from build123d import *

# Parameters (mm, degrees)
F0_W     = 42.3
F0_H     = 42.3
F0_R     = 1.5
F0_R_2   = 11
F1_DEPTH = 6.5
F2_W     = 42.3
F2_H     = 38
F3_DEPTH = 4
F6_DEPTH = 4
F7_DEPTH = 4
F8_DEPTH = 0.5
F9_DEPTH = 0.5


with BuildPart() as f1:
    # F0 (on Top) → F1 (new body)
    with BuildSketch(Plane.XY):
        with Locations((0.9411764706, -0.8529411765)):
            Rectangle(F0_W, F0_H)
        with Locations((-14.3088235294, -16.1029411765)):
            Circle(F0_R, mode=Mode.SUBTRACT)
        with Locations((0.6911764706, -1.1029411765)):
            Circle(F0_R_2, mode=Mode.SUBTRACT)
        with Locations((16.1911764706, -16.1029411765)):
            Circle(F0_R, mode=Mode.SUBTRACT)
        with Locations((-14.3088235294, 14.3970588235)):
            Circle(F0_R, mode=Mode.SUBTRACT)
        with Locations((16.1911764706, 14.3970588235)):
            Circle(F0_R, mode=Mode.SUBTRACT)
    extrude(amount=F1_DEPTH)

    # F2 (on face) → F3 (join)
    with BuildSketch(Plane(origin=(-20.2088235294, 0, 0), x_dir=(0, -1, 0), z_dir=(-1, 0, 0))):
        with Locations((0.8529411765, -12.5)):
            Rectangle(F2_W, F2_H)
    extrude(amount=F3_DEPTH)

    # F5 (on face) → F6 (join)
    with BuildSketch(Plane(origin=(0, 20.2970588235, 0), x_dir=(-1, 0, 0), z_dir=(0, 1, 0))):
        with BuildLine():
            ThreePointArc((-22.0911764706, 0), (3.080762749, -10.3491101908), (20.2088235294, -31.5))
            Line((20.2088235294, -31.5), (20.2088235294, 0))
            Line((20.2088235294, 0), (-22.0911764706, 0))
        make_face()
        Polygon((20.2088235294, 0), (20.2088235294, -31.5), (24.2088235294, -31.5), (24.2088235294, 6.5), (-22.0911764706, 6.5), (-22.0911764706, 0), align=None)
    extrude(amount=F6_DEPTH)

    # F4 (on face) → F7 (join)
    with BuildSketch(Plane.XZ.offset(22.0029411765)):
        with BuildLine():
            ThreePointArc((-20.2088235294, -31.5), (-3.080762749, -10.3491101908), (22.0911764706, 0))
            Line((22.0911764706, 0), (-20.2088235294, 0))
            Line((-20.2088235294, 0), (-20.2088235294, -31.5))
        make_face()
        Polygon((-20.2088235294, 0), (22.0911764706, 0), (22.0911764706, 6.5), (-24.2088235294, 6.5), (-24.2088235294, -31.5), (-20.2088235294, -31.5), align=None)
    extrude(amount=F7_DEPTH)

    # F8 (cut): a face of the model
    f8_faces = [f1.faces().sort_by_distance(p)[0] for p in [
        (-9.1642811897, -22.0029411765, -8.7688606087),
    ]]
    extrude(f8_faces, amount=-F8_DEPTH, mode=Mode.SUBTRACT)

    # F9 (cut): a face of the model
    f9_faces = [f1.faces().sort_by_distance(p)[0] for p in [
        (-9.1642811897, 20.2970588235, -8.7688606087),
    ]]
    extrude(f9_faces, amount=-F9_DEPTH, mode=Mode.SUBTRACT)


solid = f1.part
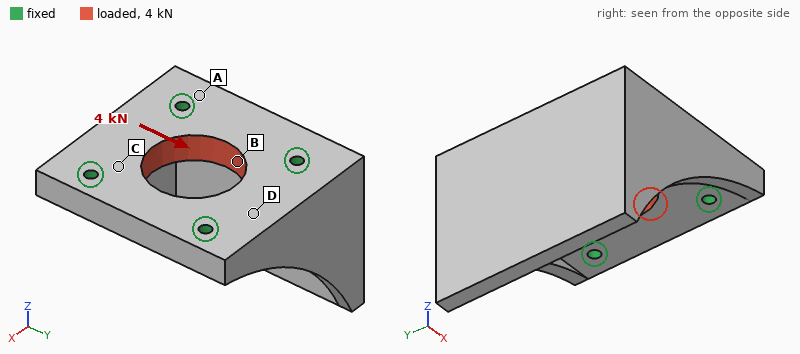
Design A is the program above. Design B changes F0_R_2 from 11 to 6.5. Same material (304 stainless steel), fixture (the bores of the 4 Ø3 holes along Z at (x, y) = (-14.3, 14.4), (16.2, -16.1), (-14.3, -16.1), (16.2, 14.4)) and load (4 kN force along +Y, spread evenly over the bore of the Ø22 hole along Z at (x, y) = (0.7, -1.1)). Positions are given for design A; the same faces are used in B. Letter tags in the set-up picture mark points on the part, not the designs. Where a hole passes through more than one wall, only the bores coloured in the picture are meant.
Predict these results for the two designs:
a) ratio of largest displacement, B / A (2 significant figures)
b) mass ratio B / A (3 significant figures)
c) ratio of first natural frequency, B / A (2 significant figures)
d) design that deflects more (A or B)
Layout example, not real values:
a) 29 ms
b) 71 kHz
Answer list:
a) 1.1
b) 1.07
c) 1.0
d) B
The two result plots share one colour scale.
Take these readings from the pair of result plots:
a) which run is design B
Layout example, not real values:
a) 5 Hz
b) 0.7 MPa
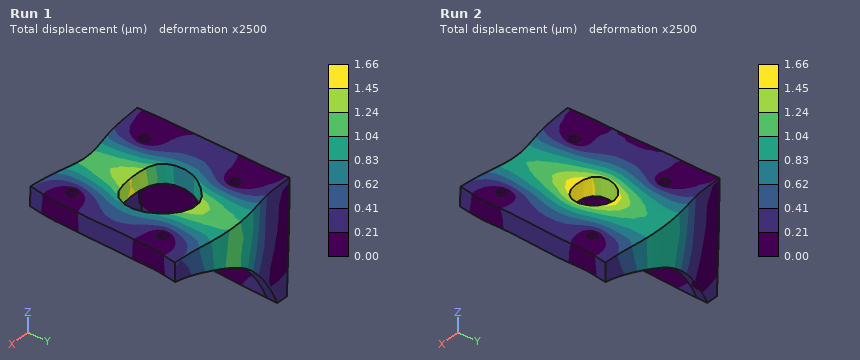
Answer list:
a) Run 2
